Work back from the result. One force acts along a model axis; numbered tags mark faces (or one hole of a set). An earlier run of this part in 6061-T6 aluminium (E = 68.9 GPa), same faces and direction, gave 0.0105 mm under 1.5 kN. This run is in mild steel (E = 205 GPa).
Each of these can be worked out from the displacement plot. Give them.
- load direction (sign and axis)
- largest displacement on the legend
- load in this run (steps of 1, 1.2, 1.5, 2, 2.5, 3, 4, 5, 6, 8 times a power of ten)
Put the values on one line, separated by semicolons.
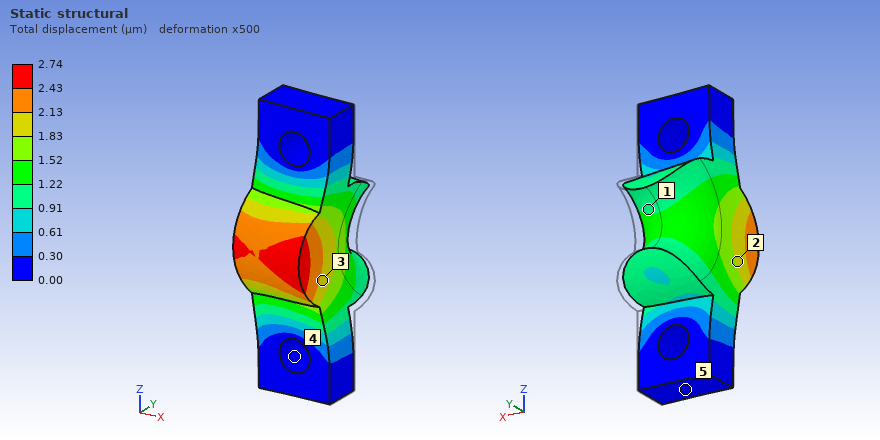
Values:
-X; 2.74 µm; 1.2 kN
